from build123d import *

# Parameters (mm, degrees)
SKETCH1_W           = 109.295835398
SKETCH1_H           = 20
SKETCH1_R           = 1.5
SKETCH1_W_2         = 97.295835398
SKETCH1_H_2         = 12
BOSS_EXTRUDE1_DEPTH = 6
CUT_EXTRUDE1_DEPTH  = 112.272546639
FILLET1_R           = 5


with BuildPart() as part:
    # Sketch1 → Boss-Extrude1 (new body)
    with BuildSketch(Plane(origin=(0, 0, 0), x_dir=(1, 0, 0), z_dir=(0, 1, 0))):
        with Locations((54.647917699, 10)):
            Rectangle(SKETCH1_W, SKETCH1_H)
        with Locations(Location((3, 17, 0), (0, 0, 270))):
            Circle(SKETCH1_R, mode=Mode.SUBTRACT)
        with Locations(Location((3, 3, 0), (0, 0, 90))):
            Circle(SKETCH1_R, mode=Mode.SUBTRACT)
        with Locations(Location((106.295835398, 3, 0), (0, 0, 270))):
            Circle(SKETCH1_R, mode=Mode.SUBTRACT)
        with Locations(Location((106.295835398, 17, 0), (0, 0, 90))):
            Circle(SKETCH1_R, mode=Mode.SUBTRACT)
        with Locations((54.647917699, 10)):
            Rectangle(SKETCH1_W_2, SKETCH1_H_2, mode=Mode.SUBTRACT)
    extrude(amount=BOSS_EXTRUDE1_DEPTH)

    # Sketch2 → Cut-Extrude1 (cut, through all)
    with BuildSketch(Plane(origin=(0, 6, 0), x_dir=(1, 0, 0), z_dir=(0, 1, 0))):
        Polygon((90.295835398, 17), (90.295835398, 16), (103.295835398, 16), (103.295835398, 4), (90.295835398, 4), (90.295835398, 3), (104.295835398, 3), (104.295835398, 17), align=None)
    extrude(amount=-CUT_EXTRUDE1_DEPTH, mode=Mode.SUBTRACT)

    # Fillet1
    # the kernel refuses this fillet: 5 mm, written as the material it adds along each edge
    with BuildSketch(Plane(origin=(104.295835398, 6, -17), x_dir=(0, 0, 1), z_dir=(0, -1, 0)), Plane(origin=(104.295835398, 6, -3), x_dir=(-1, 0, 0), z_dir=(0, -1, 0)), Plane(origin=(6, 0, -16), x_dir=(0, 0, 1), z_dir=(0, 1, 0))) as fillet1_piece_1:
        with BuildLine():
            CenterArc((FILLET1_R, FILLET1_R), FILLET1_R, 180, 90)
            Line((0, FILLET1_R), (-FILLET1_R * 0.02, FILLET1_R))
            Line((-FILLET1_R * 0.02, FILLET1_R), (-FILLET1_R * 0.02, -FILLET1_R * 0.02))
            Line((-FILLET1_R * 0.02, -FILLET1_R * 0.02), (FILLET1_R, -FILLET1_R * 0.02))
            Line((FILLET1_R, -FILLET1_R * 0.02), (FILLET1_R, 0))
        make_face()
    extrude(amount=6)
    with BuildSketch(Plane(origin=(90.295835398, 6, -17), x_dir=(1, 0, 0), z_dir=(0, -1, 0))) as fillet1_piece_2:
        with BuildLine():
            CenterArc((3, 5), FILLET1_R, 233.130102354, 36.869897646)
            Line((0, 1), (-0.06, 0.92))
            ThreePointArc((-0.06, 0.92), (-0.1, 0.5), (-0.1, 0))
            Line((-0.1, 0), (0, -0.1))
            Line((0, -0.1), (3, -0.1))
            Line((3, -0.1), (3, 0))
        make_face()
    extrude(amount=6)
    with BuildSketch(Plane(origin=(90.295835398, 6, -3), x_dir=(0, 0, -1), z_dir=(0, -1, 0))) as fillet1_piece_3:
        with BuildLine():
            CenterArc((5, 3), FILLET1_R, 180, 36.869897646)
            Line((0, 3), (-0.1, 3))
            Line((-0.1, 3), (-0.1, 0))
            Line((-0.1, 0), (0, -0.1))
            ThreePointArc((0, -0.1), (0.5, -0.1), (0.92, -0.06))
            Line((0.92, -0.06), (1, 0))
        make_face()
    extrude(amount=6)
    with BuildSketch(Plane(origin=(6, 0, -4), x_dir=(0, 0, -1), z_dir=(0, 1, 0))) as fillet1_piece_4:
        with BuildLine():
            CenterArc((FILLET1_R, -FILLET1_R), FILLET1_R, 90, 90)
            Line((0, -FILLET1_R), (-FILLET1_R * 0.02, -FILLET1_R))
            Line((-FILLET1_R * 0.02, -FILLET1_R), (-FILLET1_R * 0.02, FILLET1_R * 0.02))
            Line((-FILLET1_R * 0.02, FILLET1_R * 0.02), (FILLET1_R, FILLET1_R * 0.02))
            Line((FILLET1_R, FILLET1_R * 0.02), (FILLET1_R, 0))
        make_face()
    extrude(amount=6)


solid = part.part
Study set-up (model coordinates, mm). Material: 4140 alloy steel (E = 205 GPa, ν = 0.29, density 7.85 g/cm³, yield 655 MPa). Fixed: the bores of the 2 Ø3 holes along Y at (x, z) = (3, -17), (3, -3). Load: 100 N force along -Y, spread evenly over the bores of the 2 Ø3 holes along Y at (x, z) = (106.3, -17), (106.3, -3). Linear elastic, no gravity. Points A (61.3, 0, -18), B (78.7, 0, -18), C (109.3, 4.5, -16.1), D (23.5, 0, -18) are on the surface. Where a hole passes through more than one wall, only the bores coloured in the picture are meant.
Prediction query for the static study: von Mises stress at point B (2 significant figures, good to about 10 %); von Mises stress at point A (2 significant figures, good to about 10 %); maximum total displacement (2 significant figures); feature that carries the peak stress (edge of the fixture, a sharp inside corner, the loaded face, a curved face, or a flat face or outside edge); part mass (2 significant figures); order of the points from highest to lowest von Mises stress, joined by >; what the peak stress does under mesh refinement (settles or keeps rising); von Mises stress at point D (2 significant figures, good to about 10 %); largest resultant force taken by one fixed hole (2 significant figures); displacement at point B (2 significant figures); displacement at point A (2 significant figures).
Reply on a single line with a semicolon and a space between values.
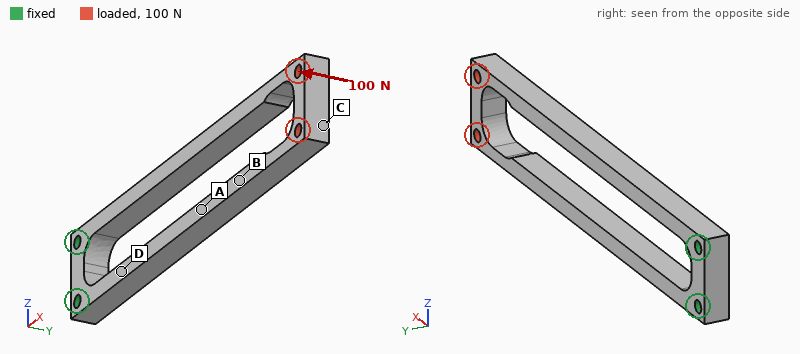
57 MPa; 94 MPa; 1.2 mm; edge of the fixture; 46 g; D > A > B > C; keeps rising; 170 MPa; 50 N; 0.71 mm; 0.45 mm
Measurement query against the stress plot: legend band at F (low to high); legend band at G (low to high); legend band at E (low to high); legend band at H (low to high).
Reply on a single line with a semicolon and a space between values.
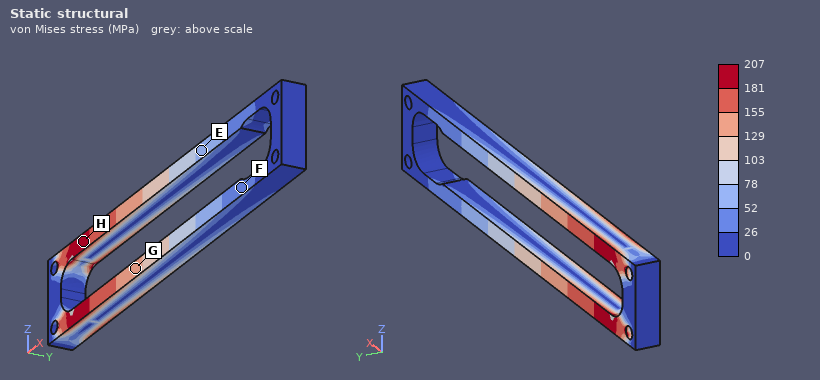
26 to 52 MPa; 129 to 155 MPa; 52 to 78 MPa; 181 to 207 MPa
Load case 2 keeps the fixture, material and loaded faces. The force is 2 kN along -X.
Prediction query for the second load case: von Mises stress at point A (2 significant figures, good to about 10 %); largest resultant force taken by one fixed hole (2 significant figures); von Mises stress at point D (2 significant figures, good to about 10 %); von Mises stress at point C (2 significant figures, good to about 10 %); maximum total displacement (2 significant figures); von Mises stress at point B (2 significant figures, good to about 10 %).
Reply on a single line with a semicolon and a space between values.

42 MPa; 1.0 kN; 42 MPa; 70 MPa; 26 µm; 42 MPa
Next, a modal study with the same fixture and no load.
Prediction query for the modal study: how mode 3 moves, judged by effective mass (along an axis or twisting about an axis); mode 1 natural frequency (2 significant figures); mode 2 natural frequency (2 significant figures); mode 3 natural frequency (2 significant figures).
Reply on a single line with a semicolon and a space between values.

twisting about X; 420 Hz; 440 Hz; 1700 Hz
